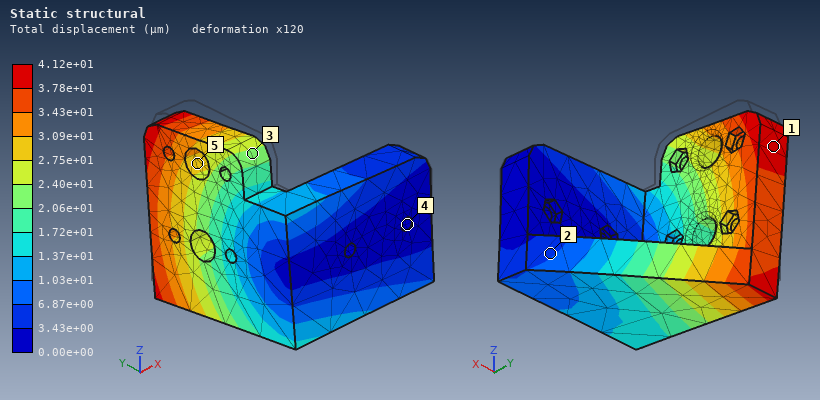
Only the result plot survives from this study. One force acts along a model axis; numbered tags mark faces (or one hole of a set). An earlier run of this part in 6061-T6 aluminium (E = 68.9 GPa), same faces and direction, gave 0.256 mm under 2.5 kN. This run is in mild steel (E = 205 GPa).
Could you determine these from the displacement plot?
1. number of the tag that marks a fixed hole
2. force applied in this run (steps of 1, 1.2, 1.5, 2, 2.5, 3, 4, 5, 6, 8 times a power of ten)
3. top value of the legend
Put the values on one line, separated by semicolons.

4; 1.2 kN; 4.12e+01 µm
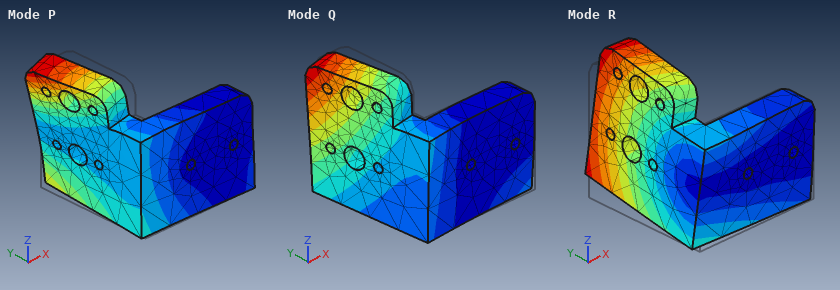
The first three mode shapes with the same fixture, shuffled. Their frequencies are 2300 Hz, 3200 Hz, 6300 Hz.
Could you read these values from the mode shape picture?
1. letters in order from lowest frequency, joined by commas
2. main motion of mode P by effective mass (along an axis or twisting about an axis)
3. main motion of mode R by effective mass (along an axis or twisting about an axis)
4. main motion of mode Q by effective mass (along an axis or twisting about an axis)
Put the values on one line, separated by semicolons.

R, Q, P; along Y; along Z; along X
